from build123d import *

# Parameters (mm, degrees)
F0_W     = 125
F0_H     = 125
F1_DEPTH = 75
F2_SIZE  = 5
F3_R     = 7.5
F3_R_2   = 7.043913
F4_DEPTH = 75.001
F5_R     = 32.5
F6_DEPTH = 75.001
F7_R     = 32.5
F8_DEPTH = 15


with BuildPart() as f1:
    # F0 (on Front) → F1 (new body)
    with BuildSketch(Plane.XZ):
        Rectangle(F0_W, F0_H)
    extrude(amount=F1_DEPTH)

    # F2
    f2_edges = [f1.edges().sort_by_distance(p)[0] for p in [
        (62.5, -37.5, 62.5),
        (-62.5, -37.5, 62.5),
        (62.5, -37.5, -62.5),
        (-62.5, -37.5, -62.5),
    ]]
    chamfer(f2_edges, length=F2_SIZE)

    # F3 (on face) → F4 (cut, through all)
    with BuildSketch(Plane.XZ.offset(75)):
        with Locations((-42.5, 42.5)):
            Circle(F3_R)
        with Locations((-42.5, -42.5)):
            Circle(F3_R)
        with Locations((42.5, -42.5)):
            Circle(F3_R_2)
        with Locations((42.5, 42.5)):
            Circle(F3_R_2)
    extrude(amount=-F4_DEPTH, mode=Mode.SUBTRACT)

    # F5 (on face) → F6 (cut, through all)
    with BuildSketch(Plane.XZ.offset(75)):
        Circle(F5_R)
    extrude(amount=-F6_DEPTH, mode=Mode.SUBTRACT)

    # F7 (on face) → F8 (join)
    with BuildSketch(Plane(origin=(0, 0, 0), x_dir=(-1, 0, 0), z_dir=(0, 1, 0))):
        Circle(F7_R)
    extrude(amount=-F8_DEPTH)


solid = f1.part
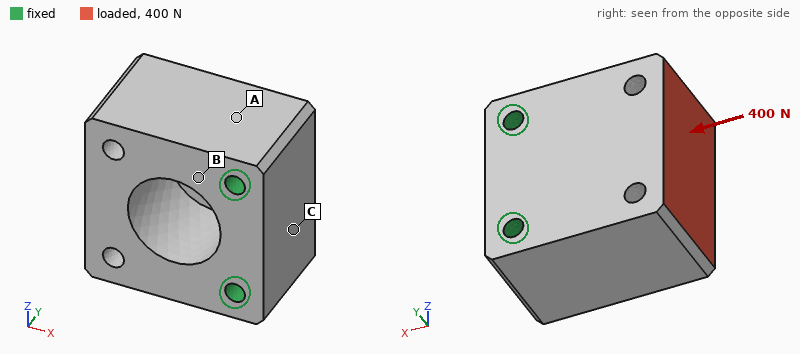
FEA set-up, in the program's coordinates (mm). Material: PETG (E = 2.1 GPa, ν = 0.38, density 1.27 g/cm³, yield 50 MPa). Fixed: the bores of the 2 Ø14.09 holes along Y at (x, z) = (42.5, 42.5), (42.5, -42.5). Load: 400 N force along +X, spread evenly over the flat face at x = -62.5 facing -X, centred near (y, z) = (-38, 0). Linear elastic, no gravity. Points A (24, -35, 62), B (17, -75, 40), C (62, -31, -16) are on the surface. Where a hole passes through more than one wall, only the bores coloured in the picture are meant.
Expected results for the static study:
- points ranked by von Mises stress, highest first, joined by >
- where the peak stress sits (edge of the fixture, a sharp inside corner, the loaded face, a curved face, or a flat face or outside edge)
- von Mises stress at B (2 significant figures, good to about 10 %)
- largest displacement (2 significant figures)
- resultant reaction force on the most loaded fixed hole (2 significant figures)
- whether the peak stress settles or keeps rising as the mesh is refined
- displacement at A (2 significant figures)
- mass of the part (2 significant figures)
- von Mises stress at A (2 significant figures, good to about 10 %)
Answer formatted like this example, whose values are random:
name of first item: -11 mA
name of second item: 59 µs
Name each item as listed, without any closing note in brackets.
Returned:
points ranked by von Mises stress, highest first, joined by >: B > A > C
where the peak stress sits: edge of the fixture
von Mises stress at B: 0.13 MPa
largest displacement: 7.5 µm
resultant reaction force on the most loaded fixed hole: 200 N
whether the peak stress settles or keeps rising as the mesh is refined: keeps rising
displacement at A: 1.3 µm
mass of the part: 1.2 kg
von Mises stress at A: 0.052 MPa
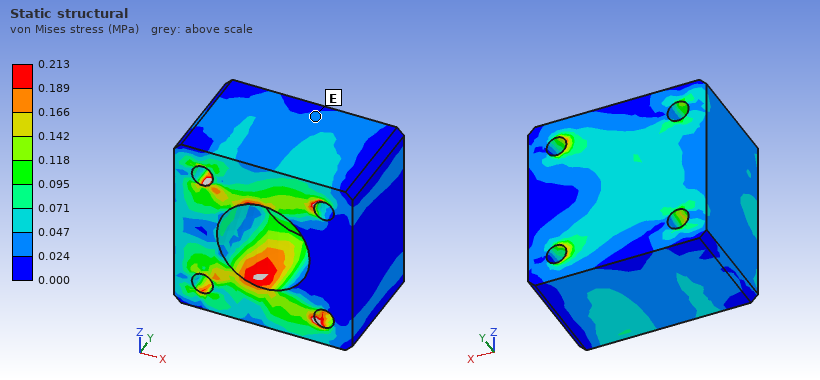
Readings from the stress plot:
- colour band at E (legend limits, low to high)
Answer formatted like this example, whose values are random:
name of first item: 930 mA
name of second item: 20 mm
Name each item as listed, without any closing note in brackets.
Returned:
colour band at E: 0.024 to 0.047 MPa
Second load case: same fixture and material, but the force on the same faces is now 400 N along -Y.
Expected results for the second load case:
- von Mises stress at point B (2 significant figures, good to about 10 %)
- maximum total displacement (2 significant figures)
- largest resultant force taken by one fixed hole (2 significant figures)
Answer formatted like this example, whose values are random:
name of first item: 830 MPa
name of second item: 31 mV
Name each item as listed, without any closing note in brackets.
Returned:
von Mises stress at point B: 0.59 MPa
maximum total displacement: 46 µm
largest resultant force taken by one fixed hole: 200 N
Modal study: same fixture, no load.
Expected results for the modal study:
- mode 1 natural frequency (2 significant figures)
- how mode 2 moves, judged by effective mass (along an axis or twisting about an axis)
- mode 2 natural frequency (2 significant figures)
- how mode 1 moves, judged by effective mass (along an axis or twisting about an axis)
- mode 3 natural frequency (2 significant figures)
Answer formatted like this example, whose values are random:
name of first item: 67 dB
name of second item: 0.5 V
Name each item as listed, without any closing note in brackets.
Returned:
mode 1 natural frequency: 890 Hz
how mode 2 moves, judged by effective mass: along Z
mode 2 natural frequency: 990 Hz
how mode 1 moves, judged by effective mass: along Y
mode 3 natural frequency: 1500 Hz
